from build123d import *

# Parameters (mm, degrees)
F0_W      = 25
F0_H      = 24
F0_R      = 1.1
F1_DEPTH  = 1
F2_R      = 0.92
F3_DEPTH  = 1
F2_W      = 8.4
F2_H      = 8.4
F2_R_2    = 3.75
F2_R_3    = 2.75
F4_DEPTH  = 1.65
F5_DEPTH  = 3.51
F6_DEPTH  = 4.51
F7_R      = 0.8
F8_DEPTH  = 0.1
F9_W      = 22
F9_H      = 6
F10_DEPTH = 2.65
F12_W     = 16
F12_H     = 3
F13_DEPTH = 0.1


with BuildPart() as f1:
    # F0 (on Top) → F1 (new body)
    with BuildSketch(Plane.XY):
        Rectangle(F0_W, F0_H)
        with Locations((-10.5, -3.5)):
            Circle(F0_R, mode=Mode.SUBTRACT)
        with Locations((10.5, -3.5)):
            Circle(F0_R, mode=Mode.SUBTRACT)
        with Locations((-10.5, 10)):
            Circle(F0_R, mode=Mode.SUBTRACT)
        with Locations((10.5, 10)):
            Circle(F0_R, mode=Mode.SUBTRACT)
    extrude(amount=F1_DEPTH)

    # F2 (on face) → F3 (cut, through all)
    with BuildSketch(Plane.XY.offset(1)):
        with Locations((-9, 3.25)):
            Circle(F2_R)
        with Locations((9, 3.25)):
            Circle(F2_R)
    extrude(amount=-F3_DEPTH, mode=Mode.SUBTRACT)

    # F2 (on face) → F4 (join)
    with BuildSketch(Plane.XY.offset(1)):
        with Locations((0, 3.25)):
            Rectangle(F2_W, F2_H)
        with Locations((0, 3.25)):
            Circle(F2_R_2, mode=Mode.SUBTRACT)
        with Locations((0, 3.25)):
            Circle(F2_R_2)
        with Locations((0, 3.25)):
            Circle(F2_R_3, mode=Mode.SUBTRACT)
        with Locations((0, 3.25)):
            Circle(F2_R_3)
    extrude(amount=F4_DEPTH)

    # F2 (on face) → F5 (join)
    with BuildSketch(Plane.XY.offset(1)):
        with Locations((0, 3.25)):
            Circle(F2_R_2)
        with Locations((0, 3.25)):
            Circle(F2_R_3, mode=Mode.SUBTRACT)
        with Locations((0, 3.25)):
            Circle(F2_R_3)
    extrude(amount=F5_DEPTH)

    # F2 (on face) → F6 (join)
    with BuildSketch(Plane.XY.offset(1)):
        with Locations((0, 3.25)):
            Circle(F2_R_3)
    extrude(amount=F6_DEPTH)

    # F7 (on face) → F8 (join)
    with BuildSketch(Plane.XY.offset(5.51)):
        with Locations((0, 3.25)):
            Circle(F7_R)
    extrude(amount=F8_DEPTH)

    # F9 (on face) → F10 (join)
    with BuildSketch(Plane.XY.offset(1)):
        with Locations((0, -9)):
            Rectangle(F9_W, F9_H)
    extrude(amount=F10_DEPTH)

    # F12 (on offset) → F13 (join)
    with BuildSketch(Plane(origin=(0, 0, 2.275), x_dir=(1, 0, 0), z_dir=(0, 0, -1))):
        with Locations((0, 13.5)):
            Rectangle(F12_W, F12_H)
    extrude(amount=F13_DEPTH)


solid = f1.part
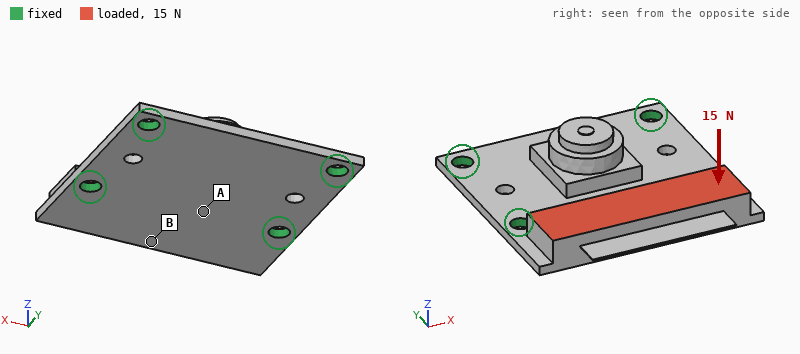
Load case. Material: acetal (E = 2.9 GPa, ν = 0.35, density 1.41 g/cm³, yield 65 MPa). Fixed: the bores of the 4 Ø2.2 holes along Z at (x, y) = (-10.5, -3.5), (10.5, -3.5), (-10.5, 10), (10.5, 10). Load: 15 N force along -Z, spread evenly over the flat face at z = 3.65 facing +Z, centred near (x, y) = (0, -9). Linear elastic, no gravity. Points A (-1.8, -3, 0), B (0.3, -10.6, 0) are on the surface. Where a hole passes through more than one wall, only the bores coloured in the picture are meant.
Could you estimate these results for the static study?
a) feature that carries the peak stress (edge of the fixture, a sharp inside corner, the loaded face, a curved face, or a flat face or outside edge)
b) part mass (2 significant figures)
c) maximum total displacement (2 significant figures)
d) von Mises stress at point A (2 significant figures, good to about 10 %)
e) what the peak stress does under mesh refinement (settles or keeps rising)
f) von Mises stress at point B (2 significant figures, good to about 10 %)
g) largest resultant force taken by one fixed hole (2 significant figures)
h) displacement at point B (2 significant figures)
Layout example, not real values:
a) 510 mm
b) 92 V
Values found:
a) edge of the fixture
b) 1.6 g
c) 0.31 mm
d) 5.9 MPa
e) keeps rising
f) 2.1 MPa
g) 9.8 N
h) 0.18 mm
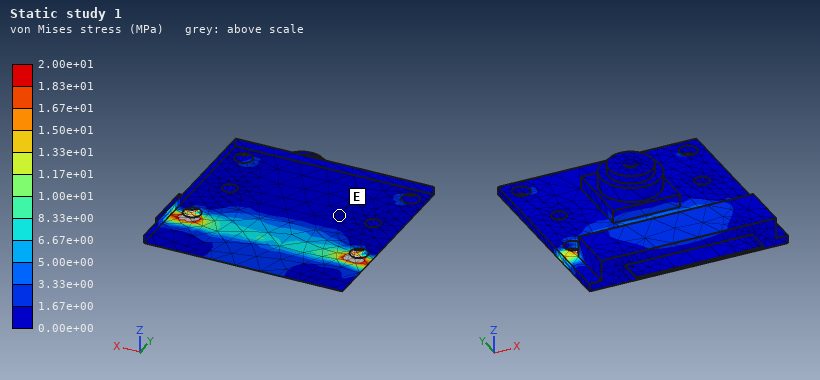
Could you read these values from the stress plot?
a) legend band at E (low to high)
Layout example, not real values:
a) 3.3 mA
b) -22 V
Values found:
a) 0.00e+00 to 1.67e+00 MPa
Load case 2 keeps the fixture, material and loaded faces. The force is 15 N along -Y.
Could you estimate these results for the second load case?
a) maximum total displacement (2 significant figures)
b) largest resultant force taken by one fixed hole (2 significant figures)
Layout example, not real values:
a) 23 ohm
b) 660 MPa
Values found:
a) 0.23 mm
b) 5.4 N
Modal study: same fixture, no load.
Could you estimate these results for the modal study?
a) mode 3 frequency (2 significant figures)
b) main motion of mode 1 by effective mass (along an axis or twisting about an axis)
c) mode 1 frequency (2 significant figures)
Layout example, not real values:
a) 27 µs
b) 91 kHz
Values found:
a) 3300 Hz
b) along Z
c) 1800 Hz
